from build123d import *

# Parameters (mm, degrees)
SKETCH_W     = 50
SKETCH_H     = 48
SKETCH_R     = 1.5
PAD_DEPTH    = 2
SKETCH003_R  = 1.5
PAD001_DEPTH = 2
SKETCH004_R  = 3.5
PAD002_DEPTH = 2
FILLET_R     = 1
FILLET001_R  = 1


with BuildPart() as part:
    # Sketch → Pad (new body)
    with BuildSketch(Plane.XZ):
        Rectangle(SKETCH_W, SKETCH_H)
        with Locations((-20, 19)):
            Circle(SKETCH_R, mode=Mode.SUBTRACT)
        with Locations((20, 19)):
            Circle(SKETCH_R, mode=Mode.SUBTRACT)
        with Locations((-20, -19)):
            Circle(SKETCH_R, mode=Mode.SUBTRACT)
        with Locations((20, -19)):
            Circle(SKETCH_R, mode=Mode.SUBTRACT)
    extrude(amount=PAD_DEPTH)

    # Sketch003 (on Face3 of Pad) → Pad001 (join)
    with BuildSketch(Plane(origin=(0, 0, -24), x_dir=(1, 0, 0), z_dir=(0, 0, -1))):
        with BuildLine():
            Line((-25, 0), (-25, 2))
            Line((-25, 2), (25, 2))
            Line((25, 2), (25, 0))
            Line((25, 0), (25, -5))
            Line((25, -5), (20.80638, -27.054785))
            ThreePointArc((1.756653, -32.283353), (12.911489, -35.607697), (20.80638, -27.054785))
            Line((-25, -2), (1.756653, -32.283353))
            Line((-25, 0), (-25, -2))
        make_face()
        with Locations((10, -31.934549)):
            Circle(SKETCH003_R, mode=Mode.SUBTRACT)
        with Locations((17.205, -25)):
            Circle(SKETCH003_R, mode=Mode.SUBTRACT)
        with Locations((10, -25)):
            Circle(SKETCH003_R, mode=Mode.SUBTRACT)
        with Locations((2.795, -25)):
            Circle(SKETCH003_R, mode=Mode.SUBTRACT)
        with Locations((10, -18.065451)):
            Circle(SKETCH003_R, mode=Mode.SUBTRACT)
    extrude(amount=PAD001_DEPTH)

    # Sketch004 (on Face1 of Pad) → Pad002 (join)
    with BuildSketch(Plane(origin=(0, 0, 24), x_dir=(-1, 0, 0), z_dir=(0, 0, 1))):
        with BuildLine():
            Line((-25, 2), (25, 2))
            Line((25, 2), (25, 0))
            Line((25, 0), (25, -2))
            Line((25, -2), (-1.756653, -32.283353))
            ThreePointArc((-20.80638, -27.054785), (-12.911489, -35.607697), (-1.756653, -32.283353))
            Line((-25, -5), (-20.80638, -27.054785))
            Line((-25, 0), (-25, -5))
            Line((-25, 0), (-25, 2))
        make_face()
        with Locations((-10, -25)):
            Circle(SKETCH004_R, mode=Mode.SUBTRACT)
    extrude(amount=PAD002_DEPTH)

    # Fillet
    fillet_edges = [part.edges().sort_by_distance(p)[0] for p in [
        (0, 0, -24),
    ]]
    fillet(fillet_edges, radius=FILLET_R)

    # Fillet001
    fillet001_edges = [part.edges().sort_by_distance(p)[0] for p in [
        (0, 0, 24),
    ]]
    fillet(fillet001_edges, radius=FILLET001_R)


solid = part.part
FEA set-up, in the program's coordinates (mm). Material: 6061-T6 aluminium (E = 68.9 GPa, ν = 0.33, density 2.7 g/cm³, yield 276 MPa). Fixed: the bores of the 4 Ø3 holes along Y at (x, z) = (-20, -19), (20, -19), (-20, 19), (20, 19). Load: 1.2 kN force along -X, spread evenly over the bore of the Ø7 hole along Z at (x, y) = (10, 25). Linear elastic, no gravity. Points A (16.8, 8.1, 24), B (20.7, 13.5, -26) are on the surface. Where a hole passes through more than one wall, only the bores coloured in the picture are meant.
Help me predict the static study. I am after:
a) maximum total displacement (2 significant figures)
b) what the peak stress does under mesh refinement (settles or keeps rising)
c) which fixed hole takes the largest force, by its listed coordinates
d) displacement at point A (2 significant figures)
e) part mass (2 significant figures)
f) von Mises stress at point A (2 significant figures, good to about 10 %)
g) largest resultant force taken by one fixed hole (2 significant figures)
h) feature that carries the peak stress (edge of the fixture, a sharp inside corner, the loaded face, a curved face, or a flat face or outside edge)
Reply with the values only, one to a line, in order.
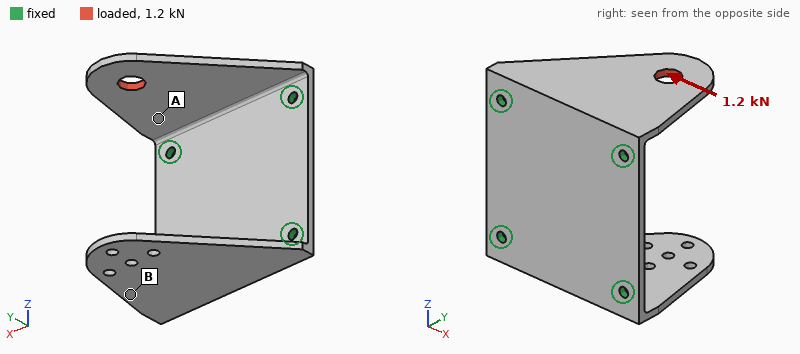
0.24 mm
keeps rising
(-20, 19)
0.096 mm
26 g
63 MPa
1.1 kN
edge of the fixture
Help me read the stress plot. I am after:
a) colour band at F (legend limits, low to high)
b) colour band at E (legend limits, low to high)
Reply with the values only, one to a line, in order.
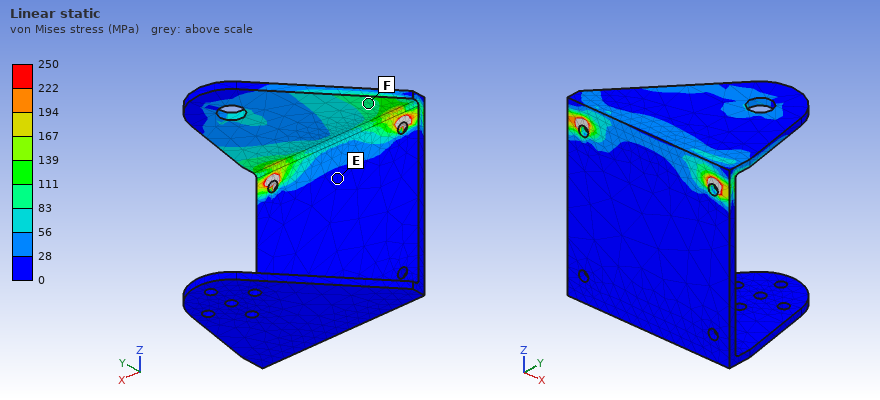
83 to 111 MPa
0 to 28 MPa
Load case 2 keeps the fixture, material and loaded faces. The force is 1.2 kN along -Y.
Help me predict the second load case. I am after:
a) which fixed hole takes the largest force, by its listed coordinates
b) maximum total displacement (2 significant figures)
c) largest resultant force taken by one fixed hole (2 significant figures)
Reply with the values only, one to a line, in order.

(20, 19)
0.45 mm
930 N
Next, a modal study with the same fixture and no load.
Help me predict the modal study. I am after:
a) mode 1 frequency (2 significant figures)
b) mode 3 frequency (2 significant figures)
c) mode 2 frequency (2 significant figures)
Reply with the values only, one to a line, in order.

1400 Hz
4500 Hz
1400 Hz
